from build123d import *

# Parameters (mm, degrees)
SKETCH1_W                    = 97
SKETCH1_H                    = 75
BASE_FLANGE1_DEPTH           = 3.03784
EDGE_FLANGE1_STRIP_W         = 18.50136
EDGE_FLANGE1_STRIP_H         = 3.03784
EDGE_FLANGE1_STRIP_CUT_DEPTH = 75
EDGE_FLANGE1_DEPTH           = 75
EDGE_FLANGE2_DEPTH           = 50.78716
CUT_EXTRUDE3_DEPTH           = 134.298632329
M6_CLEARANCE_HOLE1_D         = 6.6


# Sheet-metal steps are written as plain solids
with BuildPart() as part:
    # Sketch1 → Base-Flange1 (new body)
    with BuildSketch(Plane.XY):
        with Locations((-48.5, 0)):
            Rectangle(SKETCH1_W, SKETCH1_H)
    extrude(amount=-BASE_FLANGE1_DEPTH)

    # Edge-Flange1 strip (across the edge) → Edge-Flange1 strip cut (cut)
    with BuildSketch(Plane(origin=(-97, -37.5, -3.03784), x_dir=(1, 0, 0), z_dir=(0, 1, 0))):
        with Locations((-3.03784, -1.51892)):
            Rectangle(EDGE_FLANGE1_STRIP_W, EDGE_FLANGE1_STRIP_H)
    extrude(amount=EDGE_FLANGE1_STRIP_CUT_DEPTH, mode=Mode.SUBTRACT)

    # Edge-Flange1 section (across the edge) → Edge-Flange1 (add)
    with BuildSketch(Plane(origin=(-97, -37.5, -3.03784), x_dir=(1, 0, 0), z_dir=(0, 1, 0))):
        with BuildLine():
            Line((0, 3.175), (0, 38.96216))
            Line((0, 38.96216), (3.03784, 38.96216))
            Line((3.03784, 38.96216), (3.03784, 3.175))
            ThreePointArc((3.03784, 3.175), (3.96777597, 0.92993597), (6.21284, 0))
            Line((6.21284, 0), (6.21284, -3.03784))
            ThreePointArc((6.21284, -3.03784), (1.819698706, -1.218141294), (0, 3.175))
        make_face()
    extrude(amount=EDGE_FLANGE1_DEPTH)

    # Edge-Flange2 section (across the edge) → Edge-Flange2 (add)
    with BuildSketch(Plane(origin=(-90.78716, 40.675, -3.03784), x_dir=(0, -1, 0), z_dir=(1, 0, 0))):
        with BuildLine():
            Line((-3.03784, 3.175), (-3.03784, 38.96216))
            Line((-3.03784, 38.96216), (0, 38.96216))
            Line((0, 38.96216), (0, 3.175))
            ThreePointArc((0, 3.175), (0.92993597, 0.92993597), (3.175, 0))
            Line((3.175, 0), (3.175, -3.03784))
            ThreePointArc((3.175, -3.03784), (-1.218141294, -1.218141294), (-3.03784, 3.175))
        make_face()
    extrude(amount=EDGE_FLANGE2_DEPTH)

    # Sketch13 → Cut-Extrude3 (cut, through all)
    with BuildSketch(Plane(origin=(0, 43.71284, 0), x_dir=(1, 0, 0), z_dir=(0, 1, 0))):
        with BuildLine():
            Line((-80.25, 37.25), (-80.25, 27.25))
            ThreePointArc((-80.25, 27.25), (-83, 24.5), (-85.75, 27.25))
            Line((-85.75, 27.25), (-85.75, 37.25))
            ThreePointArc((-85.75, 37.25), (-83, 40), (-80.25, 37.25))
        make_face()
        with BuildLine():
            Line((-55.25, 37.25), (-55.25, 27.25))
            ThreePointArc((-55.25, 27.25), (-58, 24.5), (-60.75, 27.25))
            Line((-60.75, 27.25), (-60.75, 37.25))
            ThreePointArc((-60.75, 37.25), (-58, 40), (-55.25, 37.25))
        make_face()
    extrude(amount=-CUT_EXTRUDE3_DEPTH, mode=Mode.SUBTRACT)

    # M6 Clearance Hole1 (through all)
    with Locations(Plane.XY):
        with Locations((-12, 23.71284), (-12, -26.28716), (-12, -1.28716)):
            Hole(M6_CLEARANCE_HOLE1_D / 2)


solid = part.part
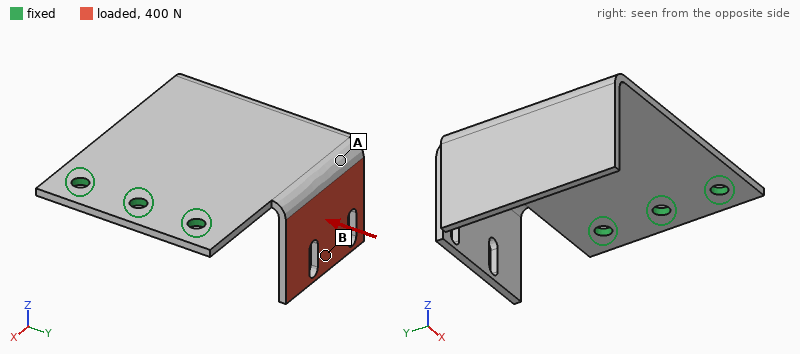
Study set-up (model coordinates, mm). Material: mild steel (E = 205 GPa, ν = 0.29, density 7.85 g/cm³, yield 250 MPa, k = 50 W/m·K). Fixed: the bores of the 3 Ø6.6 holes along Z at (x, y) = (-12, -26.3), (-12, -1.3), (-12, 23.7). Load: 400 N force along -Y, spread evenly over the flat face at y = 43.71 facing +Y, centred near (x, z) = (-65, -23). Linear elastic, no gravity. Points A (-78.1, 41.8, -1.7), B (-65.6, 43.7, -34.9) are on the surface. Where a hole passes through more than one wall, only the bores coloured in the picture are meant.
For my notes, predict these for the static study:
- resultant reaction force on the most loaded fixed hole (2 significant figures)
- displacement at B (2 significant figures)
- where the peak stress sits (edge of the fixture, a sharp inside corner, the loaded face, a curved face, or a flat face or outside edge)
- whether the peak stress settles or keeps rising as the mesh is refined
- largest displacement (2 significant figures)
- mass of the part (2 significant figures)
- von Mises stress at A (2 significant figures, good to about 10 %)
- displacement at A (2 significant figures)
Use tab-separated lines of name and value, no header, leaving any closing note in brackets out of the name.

resultant reaction force on the most loaded fixed hole	450 N
displacement at B	0.45 mm
where the peak stress sits	a sharp inside corner
whether the peak stress settles or keeps rising as the mesh is refined	keeps rising
largest displacement	0.56 mm
mass of the part	290 g
von Mises stress at A	80 MPa
displacement at A	0.22 mm
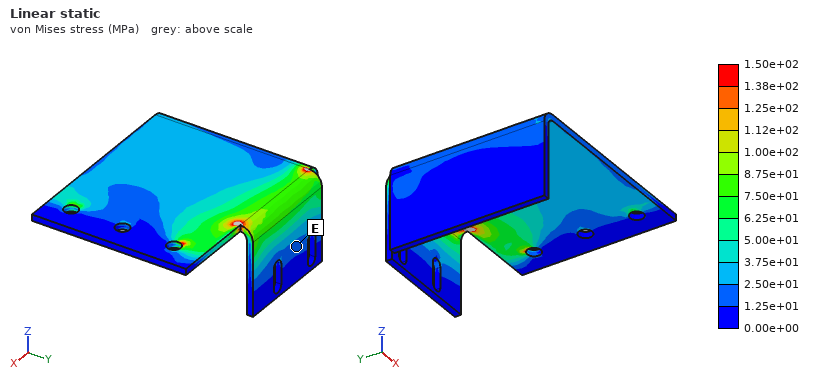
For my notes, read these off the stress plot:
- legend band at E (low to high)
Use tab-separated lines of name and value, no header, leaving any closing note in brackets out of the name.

legend band at E	1.25e+01 to 2.50e+01 MPa
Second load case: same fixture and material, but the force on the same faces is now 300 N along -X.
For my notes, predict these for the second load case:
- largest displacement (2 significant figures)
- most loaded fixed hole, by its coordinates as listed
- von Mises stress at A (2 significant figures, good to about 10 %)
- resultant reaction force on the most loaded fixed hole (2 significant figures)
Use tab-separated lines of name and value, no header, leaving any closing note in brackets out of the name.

largest displacement	0.69 mm
most loaded fixed hole, by its coordinates as listed	(-12, 23.7)
von Mises stress at A	19 MPa
resultant reaction force on the most loaded fixed hole	370 N
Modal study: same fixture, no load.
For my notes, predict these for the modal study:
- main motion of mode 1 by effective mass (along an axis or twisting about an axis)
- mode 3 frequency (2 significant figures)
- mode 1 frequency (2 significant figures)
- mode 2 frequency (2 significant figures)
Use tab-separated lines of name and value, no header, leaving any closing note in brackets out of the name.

main motion of mode 1 by effective mass	along Z
mode 3 frequency	930 Hz
mode 1 frequency	200 Hz
mode 2 frequency	430 Hz
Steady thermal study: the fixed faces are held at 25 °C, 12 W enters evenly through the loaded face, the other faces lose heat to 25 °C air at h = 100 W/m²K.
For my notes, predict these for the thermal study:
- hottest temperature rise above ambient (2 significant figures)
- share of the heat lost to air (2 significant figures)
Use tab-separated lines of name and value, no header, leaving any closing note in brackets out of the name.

hottest temperature rise above ambient	30 K
share of the heat lost to air	93 %
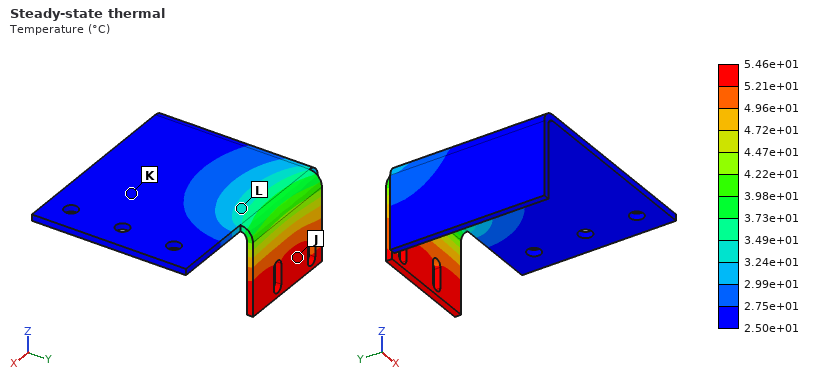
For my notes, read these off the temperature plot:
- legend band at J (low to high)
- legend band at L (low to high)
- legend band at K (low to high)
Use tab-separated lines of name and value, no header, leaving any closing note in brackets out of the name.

legend band at J	5.21e+01 to 5.46e+01 °C
legend band at L	3.24e+01 to 3.49e+01 °C
legend band at K	2.50e+01 to 2.75e+01 °C
